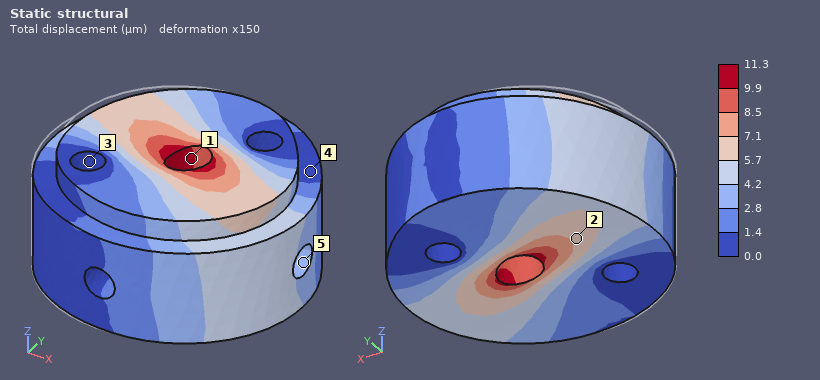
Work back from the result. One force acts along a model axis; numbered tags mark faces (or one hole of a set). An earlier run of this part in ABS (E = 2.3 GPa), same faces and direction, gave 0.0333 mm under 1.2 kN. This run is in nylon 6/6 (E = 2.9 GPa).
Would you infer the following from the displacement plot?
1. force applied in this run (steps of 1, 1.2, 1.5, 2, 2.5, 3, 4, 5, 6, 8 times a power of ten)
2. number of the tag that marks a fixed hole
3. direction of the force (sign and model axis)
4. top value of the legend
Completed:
500 N
3
+X
11.3 µm
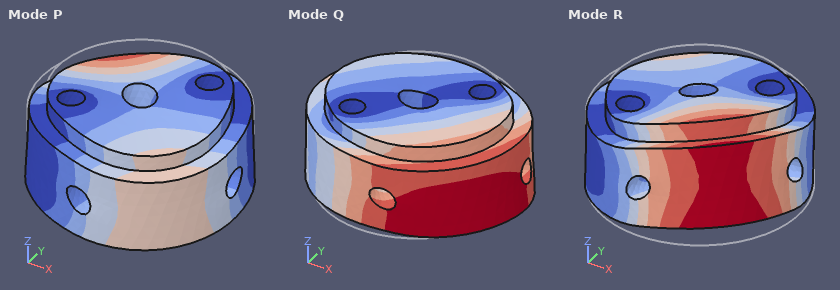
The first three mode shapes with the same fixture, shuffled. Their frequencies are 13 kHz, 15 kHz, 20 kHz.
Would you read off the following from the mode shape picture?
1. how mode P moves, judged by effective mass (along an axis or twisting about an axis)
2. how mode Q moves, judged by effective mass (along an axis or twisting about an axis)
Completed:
along Z
twisting about Z
